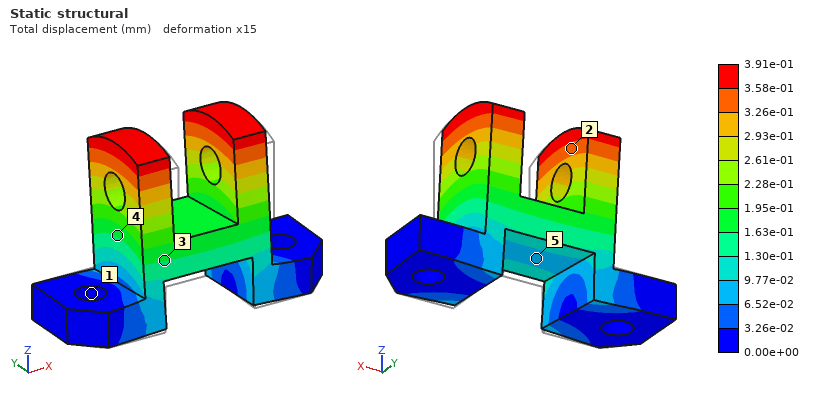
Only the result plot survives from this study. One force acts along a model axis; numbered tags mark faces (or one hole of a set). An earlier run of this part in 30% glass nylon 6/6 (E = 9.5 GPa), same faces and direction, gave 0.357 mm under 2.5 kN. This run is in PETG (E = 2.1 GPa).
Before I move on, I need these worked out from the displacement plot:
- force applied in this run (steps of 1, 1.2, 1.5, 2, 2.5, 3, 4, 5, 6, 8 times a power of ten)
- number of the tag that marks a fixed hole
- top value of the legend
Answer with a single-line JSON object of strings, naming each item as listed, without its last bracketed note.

{"force applied in this run": "600 N", "number of the tag that marks a fixed hole": "1", "top value of the legend": "3.91e-01 mm"}
